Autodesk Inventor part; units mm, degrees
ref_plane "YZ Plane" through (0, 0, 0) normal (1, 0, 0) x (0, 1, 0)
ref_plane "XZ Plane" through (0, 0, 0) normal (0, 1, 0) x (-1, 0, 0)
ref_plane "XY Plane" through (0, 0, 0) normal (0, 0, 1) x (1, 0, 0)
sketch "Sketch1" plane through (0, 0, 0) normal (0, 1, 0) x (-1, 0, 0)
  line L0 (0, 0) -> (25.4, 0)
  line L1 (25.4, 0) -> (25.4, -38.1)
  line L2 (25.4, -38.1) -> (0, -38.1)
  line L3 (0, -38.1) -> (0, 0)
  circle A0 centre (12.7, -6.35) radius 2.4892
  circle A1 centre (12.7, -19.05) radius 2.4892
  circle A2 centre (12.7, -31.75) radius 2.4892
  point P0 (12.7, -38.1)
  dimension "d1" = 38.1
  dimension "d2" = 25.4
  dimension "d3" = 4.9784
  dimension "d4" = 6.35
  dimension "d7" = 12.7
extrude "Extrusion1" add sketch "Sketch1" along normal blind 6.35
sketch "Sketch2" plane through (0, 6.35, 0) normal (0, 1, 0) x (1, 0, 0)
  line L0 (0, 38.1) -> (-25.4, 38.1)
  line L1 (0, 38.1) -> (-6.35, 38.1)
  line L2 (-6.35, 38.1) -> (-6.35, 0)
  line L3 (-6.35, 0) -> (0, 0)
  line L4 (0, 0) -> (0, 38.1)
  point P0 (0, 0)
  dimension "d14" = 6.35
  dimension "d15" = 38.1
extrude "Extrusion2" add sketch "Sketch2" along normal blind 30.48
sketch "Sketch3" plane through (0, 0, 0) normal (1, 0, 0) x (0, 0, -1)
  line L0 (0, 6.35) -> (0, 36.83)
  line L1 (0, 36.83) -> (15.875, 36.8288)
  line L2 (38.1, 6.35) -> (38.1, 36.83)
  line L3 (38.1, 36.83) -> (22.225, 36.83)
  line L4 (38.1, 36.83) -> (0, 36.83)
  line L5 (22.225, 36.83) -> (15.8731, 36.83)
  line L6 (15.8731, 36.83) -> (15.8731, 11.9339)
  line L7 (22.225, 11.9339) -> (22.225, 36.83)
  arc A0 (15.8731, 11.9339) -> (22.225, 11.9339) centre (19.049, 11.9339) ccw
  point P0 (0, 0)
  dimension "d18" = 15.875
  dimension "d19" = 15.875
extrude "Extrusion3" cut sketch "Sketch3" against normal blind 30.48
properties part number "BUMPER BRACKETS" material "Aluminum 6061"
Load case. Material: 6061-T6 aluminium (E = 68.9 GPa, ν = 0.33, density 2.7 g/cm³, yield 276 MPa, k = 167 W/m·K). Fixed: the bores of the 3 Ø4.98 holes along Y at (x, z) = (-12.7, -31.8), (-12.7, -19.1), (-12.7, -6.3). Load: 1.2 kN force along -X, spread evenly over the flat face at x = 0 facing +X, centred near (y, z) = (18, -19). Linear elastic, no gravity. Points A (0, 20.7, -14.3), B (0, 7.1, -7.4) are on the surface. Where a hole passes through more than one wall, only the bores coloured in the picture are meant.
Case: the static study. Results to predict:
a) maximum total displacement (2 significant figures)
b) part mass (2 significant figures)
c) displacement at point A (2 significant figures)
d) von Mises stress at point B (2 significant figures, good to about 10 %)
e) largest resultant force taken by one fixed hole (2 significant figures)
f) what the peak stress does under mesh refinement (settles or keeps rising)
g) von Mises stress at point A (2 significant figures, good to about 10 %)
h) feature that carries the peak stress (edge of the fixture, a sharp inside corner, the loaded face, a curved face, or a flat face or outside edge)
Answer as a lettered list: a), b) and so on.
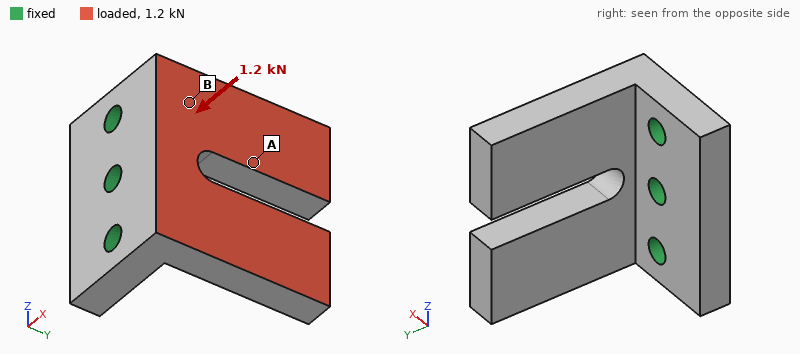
a) 0.17 mm
b) 33 g
c) 0.075 mm
d) 50 MPa
e) 410 N
f) keeps rising
g) 20 MPa
h) edge of the fixture
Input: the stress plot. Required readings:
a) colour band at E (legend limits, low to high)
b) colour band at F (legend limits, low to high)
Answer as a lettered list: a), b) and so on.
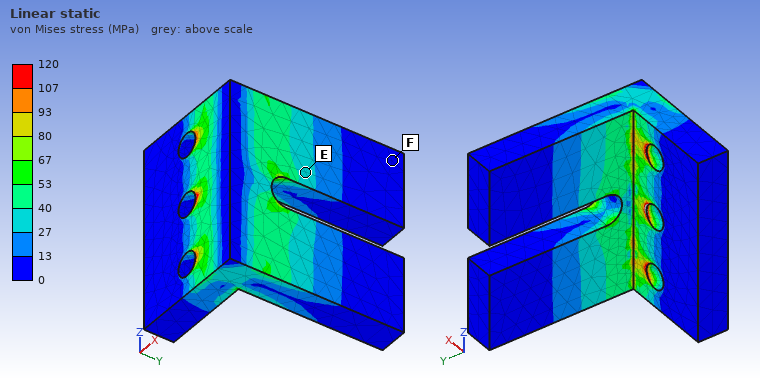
a) 27 to 40 MPa
b) 0 to 13 MPa
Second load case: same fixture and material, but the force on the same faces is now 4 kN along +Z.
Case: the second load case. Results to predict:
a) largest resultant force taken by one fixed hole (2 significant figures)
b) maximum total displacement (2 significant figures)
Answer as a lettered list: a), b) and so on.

a) 2.7 kN
b) 0.13 mm
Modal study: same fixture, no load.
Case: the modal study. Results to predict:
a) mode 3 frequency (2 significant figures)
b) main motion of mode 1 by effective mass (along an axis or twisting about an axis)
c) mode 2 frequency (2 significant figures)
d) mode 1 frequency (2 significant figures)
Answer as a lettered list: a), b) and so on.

a) 7700 Hz
b) along X
c) 4100 Hz
d) 3600 Hz
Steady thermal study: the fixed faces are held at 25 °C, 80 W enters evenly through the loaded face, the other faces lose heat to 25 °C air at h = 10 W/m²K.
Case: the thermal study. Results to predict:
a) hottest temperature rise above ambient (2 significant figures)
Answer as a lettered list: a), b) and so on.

a) 46 K
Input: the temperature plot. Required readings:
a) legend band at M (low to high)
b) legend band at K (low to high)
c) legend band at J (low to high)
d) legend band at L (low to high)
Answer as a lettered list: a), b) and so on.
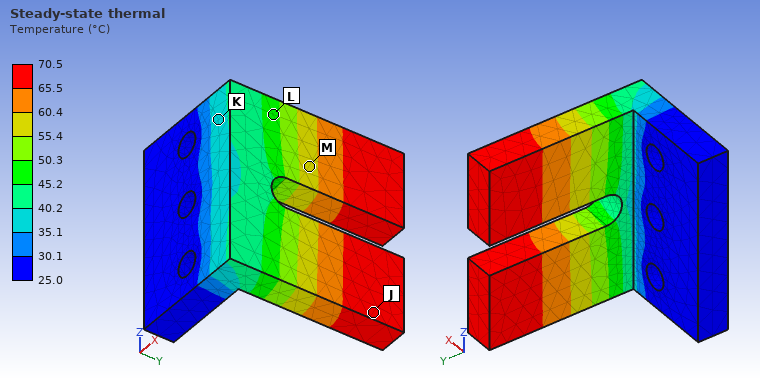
a) 55.4 to 60.4 °C
b) 35.1 to 40.2 °C
c) 65.5 to 70.5 °C
d) 45.2 to 50.3 °C
